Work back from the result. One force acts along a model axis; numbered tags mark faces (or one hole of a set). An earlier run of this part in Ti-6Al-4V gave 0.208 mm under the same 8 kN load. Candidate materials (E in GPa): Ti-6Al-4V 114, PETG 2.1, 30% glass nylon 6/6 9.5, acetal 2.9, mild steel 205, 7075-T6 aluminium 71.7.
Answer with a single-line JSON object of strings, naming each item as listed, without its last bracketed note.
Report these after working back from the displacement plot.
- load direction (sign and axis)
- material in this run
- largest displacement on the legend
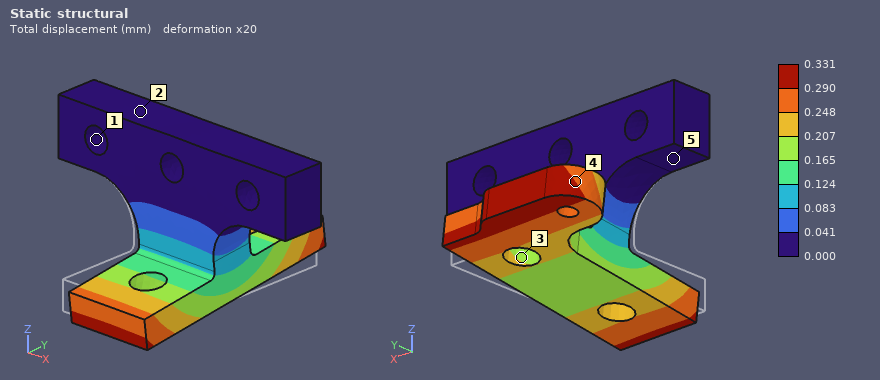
{"load direction": "+Y", "material in this run": "7075-T6 aluminium", "largest displacement on the legend": "0.331 mm"}
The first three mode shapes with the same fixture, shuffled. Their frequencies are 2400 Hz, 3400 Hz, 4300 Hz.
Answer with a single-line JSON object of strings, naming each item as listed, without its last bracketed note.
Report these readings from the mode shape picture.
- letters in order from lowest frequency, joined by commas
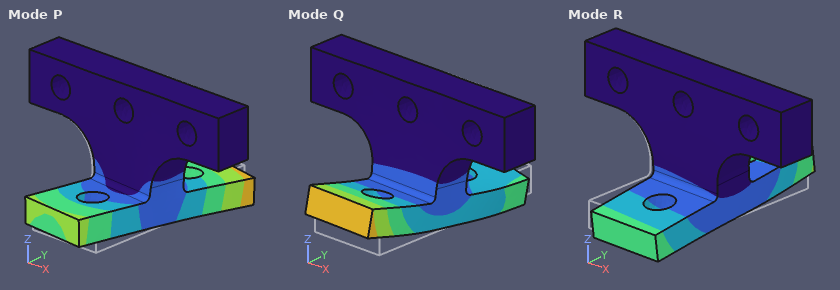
{"letters in order from lowest frequency, joined by commas": "R, P, Q"}
